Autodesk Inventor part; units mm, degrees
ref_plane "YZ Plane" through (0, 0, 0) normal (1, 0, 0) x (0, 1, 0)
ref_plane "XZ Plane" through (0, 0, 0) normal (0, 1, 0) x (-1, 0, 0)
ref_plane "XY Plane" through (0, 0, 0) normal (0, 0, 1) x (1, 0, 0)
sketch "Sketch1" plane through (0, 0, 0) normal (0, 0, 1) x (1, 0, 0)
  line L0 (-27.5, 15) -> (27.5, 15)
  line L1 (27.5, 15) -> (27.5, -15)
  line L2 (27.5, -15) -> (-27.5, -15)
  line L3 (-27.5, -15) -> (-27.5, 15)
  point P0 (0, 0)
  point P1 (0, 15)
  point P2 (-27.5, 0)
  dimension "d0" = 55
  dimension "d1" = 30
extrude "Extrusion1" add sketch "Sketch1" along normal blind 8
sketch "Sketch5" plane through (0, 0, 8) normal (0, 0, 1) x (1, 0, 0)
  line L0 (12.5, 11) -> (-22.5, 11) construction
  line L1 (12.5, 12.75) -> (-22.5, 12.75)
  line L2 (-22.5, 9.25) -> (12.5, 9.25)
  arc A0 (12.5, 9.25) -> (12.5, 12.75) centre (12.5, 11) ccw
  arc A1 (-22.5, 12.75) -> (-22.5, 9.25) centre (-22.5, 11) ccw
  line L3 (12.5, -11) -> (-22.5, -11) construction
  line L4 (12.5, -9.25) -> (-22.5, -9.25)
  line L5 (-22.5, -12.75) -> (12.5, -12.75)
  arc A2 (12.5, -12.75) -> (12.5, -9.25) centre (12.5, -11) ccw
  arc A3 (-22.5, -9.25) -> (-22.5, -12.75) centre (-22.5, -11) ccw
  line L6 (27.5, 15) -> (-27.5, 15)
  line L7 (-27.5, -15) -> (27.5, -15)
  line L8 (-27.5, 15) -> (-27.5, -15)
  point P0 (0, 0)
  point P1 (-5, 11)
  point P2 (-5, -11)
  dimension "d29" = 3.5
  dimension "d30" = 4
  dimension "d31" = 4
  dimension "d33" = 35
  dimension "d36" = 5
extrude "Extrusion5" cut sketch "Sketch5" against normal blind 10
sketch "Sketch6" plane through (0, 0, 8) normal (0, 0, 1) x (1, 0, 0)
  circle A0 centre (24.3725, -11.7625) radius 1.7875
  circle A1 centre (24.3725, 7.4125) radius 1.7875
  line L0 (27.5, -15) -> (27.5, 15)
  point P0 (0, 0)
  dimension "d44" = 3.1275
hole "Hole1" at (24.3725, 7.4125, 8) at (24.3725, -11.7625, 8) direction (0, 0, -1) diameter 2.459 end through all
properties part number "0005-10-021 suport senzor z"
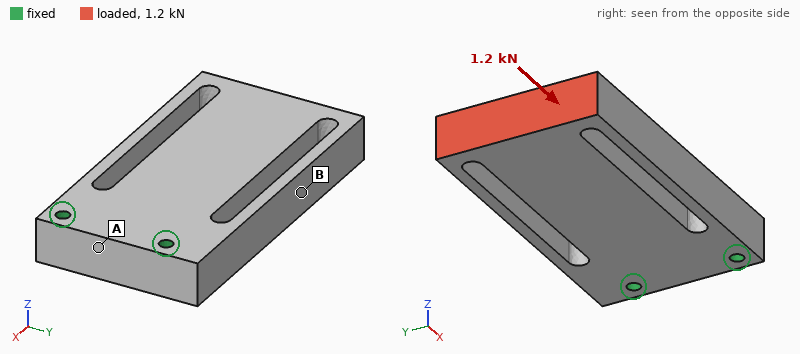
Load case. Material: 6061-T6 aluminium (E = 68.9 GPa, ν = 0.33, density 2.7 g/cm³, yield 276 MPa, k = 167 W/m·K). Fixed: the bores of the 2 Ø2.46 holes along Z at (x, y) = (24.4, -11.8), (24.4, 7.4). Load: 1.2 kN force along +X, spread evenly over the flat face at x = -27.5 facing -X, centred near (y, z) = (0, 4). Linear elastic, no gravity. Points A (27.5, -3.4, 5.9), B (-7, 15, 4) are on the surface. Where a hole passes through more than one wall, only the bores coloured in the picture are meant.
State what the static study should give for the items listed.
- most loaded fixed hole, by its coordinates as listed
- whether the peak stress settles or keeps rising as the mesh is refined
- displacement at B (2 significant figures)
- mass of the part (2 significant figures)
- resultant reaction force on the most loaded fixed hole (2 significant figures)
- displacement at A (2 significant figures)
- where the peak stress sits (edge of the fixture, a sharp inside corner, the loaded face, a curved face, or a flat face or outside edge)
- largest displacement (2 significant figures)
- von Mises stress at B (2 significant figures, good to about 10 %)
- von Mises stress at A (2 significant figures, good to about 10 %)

(24.4, 7.4)
keeps rising
4.4 µm
30 g
730 N
0.97 µm
edge of the fixture
6.0 µm
6.9 MPa
4.2 MPa
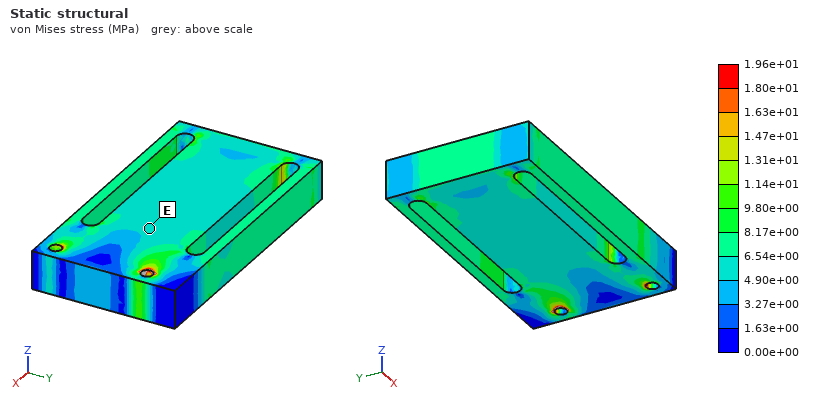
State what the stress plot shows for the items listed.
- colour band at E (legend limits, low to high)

4.90e+00 to 6.54e+00 MPa
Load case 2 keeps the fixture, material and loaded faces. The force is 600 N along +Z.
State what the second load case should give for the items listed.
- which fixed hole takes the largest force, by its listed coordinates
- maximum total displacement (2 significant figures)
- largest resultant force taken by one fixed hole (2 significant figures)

(24.4, 7.4)
0.44 mm
380 N
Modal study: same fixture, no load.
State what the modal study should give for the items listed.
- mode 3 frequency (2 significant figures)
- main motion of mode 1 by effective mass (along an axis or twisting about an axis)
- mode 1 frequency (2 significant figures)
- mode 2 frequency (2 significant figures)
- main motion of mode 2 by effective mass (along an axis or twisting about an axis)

7300 Hz
along Z
2200 Hz
5300 Hz
along Y
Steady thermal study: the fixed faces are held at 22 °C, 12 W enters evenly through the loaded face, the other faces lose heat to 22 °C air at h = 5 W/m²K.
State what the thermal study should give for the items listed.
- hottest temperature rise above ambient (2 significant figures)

20 K
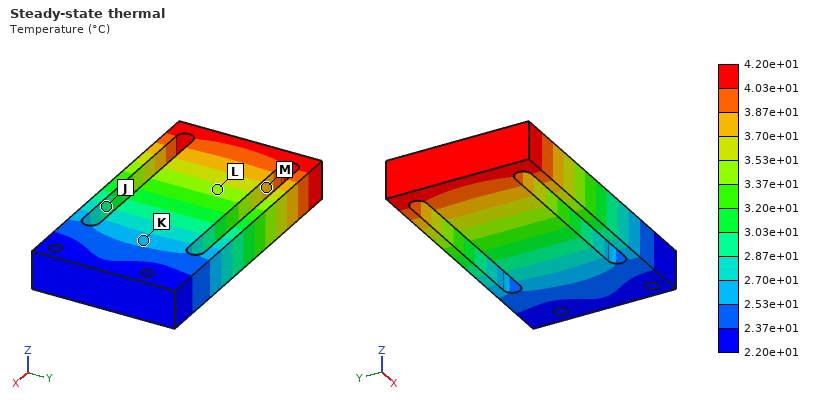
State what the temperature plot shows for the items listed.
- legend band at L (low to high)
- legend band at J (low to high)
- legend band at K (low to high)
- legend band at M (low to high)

3.37e+01 to 3.53e+01 °C
2.87e+01 to 3.03e+01 °C
2.53e+01 to 2.70e+01 °C
3.70e+01 to 3.87e+01 °C
